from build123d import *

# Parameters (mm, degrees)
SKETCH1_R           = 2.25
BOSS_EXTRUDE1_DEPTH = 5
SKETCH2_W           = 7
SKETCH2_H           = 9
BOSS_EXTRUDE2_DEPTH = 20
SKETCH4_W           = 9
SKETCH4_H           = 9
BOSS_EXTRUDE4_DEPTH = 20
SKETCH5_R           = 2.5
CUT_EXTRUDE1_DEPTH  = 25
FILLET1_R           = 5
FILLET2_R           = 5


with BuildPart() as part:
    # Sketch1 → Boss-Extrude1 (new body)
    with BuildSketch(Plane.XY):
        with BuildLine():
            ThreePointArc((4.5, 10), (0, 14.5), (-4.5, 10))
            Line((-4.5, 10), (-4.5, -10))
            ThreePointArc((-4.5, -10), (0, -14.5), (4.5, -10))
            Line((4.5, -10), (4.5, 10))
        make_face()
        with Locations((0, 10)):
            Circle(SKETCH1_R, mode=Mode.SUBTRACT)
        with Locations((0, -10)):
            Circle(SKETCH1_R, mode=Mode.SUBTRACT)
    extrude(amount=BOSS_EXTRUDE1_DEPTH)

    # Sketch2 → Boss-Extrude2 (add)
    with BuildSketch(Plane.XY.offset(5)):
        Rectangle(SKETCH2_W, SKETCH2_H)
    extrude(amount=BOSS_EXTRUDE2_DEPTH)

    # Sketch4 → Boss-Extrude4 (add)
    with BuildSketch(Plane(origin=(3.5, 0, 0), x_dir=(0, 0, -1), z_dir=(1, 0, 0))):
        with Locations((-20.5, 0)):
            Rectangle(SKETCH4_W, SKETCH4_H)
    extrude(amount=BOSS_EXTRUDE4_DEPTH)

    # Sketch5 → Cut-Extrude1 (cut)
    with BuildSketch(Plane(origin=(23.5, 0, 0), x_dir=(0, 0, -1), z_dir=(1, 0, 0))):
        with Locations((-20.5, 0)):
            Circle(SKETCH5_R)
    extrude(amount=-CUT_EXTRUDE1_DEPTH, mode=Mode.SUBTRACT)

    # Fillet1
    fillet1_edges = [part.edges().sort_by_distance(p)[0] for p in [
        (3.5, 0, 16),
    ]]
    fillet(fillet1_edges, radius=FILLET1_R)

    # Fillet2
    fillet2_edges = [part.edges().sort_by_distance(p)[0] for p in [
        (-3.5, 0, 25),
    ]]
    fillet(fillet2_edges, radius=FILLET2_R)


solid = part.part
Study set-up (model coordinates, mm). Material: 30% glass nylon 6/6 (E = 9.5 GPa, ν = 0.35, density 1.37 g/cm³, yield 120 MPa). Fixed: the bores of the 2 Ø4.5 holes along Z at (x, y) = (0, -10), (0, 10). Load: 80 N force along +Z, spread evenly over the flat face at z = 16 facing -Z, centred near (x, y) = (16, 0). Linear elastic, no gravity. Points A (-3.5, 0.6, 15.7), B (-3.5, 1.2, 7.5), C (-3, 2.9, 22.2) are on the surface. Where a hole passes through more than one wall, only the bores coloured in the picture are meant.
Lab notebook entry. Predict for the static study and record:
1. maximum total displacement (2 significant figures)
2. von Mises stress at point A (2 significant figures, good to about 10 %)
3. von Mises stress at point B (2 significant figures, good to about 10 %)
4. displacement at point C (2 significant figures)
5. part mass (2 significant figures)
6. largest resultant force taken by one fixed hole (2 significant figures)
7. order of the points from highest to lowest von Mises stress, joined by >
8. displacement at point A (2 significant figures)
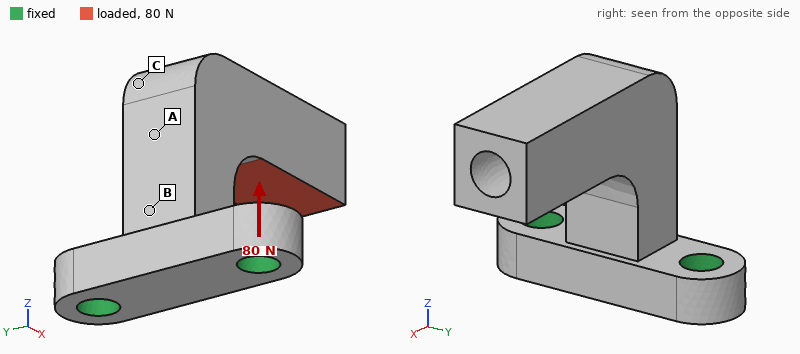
0.32 mm
9.6 MPa
15 MPa
0.15 mm
4.7 g
41 N
B > A > C
0.086 mm
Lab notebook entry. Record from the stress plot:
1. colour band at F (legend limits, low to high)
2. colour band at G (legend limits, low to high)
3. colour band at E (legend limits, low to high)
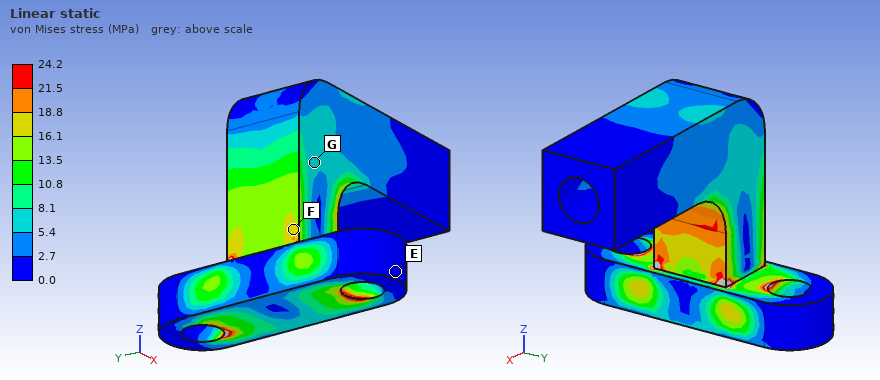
16.1 to 18.8 MPa
5.4 to 8.1 MPa
0.0 to 2.7 MPa
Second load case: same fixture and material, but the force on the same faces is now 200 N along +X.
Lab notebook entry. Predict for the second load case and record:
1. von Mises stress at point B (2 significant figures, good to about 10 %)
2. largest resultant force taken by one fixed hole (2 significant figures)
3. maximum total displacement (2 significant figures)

21 MPa
100 N
0.39 mm
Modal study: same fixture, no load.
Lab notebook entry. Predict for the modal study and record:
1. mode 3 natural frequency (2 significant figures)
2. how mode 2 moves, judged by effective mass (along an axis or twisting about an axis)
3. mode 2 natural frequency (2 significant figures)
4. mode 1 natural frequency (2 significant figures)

6400 Hz
along Y
2600 Hz
1900 Hz
